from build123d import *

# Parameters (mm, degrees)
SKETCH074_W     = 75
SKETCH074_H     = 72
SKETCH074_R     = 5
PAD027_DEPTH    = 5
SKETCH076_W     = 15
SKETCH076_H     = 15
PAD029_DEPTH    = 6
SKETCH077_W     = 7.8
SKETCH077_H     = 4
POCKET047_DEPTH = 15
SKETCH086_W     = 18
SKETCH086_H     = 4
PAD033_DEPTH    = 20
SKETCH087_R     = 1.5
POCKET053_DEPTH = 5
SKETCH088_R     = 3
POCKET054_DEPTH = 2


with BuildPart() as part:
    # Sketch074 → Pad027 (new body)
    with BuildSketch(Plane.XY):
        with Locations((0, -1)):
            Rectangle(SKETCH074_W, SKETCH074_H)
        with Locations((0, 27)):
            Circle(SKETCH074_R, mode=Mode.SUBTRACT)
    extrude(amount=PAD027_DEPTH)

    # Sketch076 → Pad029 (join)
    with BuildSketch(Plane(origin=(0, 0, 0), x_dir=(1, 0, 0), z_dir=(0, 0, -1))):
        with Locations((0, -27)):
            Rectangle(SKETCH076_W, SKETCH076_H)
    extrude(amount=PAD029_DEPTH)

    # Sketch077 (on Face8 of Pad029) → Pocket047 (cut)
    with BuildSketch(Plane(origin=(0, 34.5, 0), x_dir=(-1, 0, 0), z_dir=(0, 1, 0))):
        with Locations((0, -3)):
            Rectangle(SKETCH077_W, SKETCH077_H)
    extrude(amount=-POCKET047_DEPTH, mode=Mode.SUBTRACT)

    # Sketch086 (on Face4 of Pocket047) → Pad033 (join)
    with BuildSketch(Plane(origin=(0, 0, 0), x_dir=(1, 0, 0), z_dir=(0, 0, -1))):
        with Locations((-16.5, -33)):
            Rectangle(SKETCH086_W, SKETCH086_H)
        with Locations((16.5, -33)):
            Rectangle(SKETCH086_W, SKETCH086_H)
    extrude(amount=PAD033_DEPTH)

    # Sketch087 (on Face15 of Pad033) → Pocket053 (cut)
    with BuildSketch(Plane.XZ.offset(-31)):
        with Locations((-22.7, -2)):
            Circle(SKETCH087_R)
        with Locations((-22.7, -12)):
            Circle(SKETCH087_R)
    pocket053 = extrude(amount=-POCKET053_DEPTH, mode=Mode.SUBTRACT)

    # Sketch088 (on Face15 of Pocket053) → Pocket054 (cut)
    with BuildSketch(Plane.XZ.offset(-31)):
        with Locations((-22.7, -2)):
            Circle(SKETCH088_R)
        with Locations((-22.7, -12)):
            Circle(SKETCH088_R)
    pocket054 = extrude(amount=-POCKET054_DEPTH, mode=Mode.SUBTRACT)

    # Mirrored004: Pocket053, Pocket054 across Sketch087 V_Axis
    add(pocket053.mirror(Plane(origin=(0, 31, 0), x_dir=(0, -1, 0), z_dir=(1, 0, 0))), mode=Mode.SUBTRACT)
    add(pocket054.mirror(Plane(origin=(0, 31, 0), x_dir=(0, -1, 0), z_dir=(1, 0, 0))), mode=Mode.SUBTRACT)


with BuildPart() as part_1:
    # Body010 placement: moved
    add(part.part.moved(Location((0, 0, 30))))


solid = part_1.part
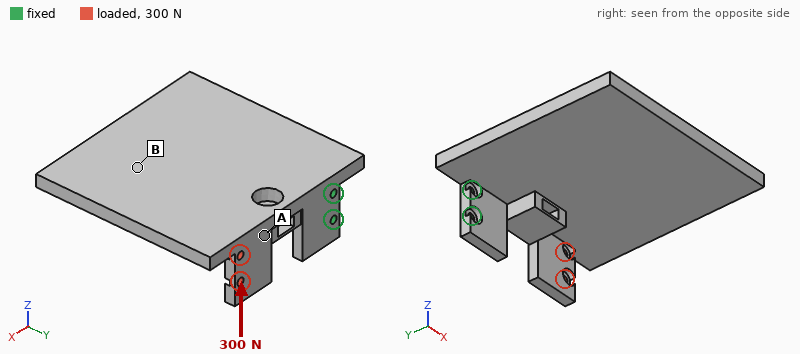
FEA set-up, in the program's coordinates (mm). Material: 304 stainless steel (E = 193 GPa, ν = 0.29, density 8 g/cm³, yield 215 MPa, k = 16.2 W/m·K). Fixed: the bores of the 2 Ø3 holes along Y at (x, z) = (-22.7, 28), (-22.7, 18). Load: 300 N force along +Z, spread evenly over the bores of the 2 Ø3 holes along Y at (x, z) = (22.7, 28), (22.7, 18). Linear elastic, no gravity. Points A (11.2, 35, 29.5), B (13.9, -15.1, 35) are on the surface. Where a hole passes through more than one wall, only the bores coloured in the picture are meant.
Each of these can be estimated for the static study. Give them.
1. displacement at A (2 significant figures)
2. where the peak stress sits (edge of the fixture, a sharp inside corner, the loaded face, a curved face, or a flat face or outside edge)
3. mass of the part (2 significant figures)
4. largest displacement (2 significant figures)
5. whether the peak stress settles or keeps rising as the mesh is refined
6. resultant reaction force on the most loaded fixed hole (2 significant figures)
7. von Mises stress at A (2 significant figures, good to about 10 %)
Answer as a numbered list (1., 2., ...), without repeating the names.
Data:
1. 40 µm
2. edge of the fixture
3. 240 g
4. 88 µm
5. keeps rising
6. 1.1 kN
7. 23 MPa
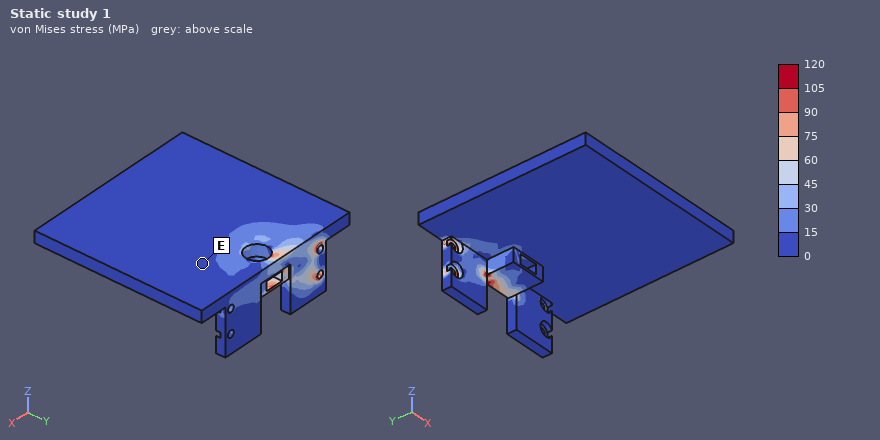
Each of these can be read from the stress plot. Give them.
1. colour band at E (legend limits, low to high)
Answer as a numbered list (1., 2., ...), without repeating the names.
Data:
1. 0 to 15 MPa
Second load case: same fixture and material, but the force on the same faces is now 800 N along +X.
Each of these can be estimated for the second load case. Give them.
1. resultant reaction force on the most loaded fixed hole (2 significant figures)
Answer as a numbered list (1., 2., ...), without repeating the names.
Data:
1. 420 N
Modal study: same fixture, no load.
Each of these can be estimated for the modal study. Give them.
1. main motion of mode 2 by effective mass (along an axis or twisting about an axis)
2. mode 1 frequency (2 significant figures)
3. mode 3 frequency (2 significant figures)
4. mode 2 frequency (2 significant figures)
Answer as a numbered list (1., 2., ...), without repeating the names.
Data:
1. along Z
2. 280 Hz
3. 1100 Hz
4. 390 Hz
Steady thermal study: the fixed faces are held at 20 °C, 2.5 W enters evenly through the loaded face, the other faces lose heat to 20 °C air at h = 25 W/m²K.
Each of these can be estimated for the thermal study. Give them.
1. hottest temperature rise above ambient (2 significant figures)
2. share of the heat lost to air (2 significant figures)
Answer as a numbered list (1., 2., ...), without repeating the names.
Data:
1. 42 K
2. 87 %
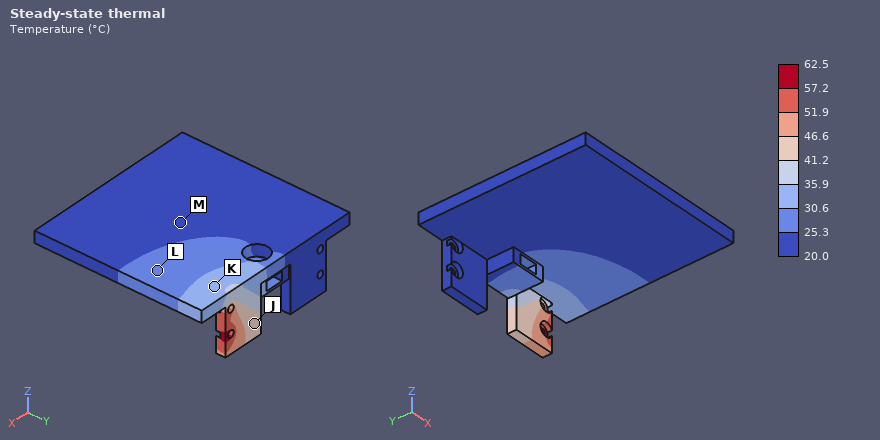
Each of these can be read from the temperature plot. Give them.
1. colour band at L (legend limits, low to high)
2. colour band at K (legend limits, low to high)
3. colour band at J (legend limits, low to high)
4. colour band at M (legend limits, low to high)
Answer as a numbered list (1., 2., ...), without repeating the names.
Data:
1. 25.3 to 30.6 °C
2. 30.6 to 35.9 °C
3. 41.2 to 46.6 °C
4. 20.0 to 25.3 °C
